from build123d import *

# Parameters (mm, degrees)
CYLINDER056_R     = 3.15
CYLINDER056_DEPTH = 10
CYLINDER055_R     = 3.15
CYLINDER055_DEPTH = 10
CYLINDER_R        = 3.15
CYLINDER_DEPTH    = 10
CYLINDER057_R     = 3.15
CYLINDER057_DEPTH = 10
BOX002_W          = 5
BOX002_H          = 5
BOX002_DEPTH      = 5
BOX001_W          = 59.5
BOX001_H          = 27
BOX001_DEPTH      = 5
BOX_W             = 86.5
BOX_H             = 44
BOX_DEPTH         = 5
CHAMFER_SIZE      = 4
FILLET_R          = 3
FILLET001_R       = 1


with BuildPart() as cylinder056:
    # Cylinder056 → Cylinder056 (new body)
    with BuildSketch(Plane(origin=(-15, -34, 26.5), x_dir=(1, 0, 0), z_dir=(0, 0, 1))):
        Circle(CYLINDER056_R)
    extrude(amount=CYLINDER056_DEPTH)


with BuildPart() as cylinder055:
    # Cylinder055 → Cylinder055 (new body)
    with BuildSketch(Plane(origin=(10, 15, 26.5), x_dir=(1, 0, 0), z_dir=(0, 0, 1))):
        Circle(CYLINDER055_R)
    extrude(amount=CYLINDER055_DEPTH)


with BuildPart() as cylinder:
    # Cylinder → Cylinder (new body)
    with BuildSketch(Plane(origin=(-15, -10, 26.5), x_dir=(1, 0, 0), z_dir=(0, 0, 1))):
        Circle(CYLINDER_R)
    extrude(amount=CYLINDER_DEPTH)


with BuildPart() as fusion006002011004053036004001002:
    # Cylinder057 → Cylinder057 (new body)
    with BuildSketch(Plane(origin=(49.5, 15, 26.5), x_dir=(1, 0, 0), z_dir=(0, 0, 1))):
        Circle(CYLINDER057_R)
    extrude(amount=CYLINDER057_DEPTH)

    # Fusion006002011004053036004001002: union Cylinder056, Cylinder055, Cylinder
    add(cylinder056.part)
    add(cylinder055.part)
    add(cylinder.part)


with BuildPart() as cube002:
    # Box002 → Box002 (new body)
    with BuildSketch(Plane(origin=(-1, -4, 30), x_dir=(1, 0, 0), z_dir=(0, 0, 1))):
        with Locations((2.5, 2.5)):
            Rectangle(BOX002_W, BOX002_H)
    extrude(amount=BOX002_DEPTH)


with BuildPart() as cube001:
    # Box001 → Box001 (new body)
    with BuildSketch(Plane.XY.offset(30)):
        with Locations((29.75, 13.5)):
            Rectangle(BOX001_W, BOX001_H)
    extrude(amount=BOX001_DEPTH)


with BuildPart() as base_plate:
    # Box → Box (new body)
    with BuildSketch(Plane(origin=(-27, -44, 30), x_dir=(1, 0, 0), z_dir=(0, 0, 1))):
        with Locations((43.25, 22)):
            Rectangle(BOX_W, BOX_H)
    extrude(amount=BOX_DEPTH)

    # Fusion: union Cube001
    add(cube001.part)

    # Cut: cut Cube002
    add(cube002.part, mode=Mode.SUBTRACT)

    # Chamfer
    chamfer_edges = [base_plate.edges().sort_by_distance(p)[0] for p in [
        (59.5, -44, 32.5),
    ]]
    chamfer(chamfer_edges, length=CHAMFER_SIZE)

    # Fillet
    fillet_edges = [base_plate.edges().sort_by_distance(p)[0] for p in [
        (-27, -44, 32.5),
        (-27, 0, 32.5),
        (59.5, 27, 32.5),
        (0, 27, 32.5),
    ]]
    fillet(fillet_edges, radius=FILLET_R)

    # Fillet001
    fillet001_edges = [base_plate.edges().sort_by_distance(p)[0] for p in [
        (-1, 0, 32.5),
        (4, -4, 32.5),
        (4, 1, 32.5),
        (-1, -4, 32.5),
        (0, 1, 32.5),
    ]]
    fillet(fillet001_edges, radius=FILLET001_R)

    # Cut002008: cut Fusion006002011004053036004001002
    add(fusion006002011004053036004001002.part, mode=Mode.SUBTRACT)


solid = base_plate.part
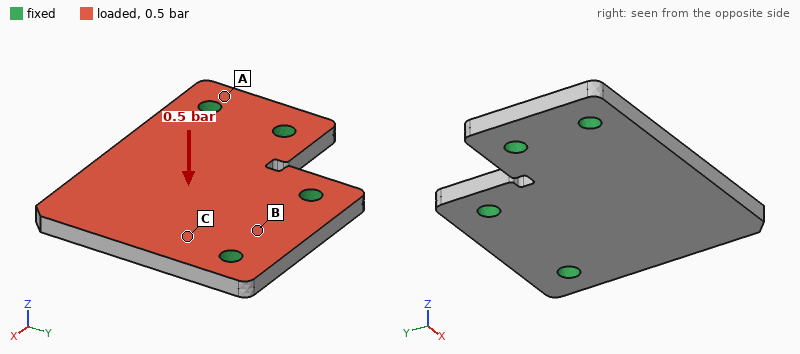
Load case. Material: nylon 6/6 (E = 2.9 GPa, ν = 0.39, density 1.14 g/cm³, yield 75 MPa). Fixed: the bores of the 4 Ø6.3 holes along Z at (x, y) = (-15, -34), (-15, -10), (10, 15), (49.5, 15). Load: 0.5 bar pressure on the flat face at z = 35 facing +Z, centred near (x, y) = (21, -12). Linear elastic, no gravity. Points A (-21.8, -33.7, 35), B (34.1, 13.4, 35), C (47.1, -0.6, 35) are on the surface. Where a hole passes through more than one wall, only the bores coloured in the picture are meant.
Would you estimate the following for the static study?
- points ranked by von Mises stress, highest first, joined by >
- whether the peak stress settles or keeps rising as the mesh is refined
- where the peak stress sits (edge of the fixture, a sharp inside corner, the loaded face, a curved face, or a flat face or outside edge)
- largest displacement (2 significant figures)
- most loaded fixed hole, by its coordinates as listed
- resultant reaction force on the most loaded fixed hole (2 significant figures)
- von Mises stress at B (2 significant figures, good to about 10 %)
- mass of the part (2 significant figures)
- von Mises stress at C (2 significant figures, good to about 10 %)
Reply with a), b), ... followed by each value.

a) C > B > A
b) keeps rising
c) edge of the fixture
d) 1.2 mm
e) (49.5, 15)
f) 100 N
g) 3.4 MPa
h) 30 g
i) 5.0 MPa
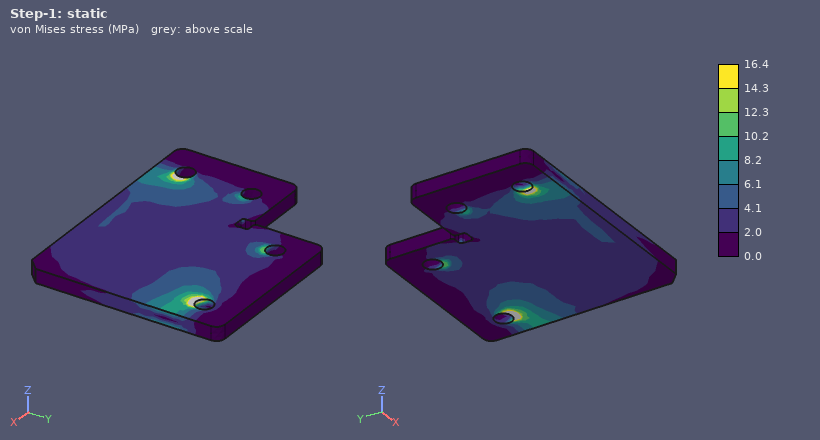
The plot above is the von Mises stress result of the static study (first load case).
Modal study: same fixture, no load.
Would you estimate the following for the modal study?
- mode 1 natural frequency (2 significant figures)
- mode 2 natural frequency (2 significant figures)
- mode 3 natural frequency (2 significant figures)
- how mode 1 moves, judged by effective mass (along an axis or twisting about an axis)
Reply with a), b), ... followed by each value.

a) 620 Hz
b) 1800 Hz
c) 2500 Hz
d) along Z
